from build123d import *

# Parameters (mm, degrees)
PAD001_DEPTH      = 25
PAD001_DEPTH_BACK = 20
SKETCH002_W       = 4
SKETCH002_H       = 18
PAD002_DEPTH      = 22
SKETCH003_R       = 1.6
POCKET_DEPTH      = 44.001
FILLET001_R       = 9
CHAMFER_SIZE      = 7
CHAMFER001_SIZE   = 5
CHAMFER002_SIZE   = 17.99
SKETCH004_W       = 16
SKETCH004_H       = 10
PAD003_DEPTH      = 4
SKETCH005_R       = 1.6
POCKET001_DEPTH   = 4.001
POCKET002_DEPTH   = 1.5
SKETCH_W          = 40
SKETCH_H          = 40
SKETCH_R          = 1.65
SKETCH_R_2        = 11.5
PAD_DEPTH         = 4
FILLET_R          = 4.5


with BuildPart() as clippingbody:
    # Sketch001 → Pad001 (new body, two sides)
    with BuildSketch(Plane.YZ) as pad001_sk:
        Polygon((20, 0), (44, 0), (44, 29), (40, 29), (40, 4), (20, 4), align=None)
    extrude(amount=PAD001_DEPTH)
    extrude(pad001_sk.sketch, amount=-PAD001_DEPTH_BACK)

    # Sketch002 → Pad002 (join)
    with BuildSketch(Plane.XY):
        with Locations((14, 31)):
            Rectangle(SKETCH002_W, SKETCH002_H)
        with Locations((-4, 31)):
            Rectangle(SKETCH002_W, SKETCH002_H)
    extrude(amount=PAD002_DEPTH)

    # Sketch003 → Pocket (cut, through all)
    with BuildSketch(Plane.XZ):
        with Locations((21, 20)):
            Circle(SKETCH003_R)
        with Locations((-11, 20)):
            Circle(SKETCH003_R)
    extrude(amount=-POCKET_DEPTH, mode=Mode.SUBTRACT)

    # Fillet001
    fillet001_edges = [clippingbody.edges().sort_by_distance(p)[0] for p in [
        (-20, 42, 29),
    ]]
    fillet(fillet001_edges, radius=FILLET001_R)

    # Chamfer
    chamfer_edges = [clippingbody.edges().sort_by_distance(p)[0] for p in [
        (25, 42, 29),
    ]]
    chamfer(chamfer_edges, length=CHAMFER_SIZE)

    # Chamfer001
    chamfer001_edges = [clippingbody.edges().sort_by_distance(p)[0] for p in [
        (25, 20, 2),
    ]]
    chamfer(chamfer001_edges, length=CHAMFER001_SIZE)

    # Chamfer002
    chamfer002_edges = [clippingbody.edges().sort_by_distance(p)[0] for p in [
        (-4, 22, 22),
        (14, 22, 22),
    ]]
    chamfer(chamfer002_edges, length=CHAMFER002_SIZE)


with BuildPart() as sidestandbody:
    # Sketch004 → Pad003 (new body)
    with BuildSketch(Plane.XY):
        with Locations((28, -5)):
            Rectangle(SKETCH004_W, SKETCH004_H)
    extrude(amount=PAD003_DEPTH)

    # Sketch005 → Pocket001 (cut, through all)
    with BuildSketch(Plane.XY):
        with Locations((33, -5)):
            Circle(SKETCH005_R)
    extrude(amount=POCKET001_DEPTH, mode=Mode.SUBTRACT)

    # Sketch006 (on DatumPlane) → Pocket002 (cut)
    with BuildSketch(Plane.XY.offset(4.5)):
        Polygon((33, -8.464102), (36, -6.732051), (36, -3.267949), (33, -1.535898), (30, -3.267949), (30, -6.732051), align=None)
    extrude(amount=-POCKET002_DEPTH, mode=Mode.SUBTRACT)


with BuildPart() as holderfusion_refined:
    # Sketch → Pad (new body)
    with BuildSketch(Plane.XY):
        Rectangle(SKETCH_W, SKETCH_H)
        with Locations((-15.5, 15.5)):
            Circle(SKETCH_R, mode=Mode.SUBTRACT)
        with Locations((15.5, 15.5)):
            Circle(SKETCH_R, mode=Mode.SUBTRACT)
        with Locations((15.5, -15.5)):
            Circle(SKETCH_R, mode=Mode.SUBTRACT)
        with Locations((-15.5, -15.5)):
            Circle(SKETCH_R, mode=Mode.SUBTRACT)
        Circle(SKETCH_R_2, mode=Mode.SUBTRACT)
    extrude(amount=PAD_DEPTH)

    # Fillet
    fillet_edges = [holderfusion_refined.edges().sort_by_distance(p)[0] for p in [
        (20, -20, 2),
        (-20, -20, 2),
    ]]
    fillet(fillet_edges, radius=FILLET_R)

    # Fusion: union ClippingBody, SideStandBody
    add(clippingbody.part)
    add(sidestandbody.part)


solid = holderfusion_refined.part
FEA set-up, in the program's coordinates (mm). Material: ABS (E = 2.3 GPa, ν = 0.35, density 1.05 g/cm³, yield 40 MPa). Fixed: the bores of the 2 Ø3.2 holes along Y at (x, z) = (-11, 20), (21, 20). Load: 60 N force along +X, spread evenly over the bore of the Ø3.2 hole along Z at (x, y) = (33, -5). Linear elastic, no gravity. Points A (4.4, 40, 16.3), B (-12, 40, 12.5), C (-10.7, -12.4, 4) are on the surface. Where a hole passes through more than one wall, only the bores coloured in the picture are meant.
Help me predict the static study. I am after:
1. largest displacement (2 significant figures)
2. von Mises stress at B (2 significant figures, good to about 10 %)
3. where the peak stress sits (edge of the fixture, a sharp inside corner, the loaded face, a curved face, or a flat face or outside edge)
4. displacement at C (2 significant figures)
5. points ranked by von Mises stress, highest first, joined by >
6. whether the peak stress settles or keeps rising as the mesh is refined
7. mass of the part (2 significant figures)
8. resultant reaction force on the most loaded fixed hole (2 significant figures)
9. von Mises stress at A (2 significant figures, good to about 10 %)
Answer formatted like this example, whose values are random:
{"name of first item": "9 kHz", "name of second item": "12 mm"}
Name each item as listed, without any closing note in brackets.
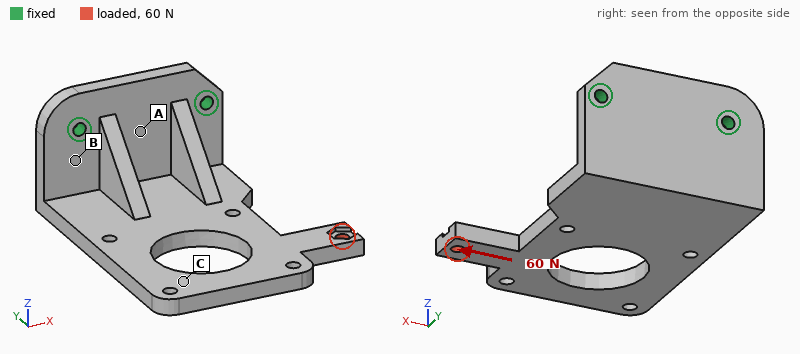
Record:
{"largest displacement": "0.92 mm", "von Mises stress at B": "4.7 MPa", "where the peak stress sits": "edge of the fixture", "displacement at C": "0.79 mm", "points ranked by von Mises stress, highest first, joined by >": "B > A > C", "whether the peak stress settles or keeps rising as the mesh is refined": "keeps rising", "mass of the part": "16 g", "resultant reaction force on the most loaded fixed hole": "100 N", "von Mises stress at A": "3.3 MPa"}
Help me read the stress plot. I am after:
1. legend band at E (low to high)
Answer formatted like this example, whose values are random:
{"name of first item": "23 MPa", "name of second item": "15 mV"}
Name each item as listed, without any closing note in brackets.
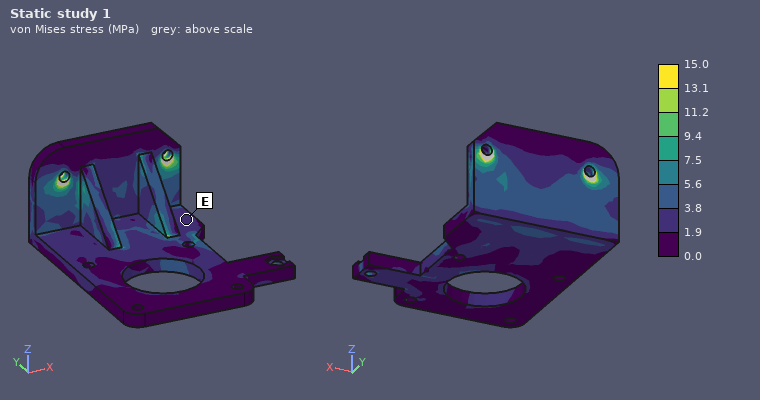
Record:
{"legend band at E": "1.9 to 3.8 MPa"}
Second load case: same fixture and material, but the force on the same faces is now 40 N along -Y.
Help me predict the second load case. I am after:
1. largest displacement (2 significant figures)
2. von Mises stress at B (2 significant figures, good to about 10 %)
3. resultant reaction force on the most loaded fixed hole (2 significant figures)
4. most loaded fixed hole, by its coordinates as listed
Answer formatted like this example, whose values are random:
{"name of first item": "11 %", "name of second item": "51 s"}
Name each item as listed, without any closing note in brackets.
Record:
{"largest displacement": "0.95 mm", "von Mises stress at B": "2.3 MPa", "resultant reaction force on the most loaded fixed hole": "57 N", "most loaded fixed hole, by its coordinates as listed": "(21, 20)"}
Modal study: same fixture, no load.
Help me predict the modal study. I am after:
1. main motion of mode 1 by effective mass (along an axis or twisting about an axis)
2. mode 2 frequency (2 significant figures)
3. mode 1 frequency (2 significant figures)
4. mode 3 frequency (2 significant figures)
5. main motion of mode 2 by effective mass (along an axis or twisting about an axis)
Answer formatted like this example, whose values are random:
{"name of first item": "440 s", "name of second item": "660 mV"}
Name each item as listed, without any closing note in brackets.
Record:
{"main motion of mode 1 by effective mass": "along Z", "mode 2 frequency": "570 Hz", "mode 1 frequency": "290 Hz", "mode 3 frequency": "760 Hz", "main motion of mode 2 by effective mass": "along X"}
